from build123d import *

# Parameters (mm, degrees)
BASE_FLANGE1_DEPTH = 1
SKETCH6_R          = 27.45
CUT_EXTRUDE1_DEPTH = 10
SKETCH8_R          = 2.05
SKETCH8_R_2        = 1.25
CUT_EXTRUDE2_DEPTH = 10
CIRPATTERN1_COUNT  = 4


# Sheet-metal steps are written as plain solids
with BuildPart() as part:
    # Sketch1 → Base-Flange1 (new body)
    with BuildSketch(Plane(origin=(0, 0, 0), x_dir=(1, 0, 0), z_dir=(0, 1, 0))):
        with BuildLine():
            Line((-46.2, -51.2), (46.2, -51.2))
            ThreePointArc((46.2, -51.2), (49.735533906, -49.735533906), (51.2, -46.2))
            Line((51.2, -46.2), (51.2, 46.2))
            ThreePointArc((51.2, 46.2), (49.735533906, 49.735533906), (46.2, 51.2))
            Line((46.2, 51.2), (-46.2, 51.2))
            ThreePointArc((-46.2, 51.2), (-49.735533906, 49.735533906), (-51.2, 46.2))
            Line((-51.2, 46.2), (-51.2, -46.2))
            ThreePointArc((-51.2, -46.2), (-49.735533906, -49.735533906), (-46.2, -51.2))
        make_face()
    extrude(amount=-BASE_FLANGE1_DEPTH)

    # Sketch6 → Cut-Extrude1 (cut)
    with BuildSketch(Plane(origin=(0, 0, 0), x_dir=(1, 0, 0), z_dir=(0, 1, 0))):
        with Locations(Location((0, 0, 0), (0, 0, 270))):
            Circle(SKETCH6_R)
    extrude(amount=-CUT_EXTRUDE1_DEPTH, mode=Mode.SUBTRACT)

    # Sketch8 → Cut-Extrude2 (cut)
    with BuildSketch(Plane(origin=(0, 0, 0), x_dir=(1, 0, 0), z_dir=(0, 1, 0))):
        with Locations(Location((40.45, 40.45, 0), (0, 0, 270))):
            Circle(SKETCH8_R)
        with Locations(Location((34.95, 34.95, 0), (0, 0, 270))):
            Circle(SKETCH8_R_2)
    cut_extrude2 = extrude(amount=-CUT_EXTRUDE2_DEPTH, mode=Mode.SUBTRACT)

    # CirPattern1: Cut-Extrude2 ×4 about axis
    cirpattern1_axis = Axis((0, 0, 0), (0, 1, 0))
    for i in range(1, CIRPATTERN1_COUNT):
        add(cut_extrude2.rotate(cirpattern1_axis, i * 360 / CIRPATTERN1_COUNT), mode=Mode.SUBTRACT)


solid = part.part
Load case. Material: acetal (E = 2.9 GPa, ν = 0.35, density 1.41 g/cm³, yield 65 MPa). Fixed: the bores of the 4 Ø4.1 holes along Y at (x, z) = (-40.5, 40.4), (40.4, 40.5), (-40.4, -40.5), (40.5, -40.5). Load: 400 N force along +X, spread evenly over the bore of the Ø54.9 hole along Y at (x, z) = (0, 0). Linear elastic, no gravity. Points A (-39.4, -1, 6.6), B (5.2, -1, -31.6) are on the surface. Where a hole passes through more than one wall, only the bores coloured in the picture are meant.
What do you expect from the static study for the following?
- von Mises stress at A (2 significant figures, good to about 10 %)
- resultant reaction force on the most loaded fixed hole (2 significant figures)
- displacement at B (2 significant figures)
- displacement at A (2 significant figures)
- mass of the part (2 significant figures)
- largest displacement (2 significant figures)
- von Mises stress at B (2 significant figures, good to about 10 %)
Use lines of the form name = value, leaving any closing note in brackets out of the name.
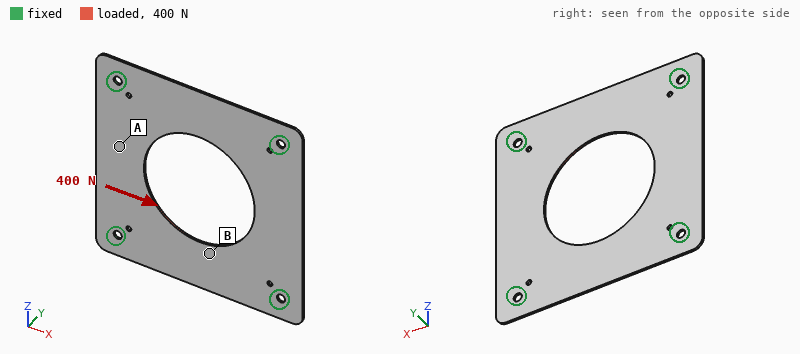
von Mises stress at A = 2.1 MPa
resultant reaction force on the most loaded fixed hole = 100 N
displacement at B = 0.050 mm
displacement at A = 0.11 mm
mass of the part = 11 g
largest displacement = 0.12 mm
von Mises stress at B = 4.7 MPa
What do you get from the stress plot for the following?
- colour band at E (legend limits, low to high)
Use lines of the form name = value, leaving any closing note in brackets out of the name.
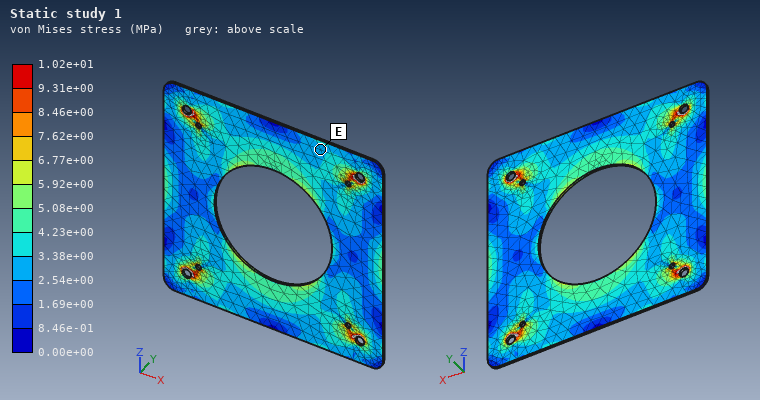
colour band at E = 2.54e+00 to 3.38e+00 MPa
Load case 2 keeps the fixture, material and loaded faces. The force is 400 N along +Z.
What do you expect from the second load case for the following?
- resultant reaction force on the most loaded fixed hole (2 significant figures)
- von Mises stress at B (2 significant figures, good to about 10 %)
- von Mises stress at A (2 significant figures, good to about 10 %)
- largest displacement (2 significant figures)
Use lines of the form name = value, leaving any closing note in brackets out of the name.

resultant reaction force on the most loaded fixed hole = 100 N
von Mises stress at B = 2.2 MPa
von Mises stress at A = 3.6 MPa
largest displacement = 0.12 mm
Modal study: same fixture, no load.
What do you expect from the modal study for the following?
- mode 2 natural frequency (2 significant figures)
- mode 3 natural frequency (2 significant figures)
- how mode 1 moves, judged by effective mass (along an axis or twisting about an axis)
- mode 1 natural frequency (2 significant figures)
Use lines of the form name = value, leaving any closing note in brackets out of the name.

mode 2 natural frequency = 250 Hz
mode 3 natural frequency = 250 Hz
how mode 1 moves, judged by effective mass = along Y
mode 1 natural frequency = 210 Hz
